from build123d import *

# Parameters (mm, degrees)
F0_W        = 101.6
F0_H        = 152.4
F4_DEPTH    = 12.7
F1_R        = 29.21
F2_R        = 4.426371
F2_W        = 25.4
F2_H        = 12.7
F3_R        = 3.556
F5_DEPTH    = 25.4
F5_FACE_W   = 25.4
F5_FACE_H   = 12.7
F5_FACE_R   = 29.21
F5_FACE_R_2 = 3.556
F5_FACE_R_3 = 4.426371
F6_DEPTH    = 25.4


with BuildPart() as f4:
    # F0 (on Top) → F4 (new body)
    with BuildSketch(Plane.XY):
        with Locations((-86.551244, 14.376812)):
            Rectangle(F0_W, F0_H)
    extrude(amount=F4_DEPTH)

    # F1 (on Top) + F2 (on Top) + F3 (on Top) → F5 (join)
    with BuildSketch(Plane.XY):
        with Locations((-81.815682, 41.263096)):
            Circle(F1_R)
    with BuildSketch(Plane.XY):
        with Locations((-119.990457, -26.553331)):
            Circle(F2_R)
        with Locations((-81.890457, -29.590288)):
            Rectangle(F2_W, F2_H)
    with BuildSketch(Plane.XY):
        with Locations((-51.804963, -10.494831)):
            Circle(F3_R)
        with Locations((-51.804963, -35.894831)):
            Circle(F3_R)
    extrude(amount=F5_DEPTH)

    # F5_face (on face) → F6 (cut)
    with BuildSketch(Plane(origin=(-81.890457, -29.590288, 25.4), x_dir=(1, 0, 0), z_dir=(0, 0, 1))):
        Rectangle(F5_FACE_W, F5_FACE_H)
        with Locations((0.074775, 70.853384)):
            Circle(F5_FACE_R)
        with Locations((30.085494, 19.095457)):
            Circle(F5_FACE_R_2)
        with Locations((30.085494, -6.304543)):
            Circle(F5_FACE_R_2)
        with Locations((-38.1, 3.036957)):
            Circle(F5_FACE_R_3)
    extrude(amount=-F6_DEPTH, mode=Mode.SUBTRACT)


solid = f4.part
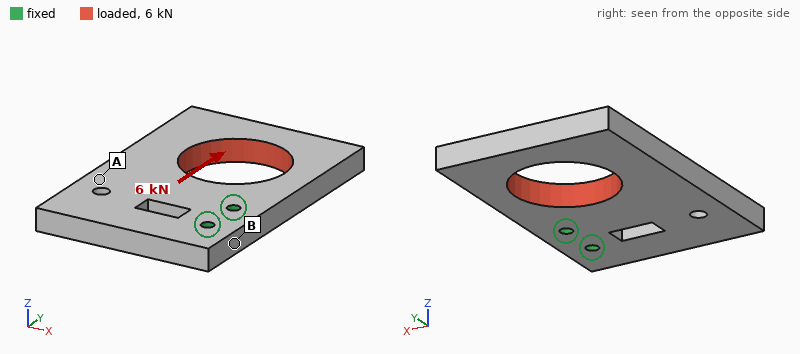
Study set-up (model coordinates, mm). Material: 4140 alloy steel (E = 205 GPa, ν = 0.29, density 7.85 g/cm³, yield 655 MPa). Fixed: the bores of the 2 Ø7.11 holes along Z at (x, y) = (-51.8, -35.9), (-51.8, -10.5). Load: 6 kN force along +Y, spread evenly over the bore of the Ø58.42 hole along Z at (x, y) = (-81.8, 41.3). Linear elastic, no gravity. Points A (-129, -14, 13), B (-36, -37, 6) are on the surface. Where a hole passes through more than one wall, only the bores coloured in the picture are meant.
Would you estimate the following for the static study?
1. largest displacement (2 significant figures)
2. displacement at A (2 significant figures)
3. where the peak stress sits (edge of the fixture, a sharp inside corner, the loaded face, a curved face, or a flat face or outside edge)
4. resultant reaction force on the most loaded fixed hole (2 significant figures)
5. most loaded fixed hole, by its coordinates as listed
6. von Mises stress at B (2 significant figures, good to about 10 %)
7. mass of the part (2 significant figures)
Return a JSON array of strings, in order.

["28 µm", "18 µm", "edge of the fixture", "6.7 kN", "(-51.8, -10.5)", "18 MPa", "1.2 kg"]
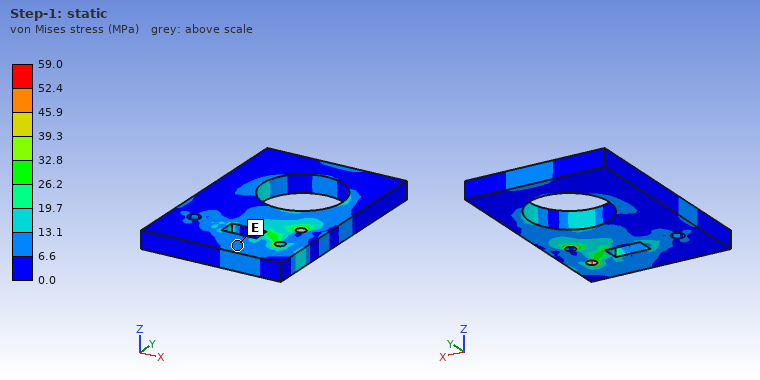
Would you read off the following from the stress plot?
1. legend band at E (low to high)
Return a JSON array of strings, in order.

["6.6 to 13.1 MPa"]
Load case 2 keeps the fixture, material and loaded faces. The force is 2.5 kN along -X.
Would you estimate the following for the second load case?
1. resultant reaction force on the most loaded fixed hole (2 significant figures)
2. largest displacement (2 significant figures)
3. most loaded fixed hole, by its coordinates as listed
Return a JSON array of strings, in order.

["6.3 kN", "31 µm", "(-51.8, -10.5)"]
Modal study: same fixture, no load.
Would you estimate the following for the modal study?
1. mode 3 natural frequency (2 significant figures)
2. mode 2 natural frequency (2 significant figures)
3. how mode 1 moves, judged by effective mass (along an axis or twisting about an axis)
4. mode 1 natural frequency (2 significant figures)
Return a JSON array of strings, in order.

["1700 Hz", "1100 Hz", "along Z", "650 Hz"]
